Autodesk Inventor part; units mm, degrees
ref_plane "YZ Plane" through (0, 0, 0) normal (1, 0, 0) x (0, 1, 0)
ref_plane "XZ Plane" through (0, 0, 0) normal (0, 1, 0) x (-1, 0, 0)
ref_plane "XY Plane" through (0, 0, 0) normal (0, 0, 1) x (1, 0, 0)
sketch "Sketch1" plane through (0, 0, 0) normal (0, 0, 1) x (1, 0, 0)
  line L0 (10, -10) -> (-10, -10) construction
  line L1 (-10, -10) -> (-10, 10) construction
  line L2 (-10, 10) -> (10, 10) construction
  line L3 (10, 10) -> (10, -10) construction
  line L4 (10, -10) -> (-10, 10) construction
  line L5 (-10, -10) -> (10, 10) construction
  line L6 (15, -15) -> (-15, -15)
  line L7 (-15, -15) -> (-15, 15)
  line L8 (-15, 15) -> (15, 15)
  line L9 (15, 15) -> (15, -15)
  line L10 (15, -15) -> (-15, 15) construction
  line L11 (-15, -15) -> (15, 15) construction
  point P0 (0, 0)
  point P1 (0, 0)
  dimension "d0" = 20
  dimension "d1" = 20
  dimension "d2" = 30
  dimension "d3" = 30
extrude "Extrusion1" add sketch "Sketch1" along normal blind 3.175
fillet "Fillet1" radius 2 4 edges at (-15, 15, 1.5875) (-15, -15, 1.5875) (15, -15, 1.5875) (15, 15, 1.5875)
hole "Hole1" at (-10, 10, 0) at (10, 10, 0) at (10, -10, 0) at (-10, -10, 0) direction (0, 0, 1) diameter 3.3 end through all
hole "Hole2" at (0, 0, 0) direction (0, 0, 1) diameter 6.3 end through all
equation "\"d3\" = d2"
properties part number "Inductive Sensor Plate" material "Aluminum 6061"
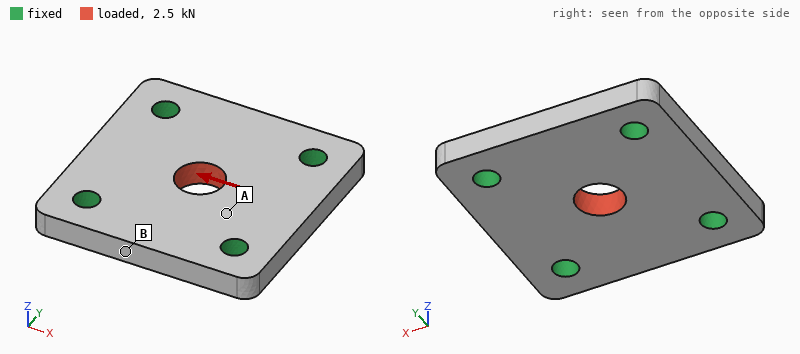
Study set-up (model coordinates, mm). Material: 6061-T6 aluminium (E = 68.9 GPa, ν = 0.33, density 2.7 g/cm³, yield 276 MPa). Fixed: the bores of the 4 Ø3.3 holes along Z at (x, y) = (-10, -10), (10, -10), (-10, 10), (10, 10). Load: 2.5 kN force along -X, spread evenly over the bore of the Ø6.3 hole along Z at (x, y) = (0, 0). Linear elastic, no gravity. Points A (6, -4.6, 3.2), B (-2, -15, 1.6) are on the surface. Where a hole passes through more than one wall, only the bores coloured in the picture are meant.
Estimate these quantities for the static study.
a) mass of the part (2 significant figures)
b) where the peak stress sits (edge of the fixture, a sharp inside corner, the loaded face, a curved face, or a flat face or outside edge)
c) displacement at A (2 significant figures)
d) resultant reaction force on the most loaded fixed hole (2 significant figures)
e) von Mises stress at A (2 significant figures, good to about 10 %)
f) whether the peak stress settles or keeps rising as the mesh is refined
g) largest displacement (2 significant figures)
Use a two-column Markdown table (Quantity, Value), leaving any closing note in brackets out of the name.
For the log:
| Quantity | Value |
|---|---|
| mass of the part | 7.1 g |
| where the peak stress sits | edge of the fixture |
| displacement at A | 3.3 µm |
| resultant reaction force on the most loaded fixed hole | 680 N |
| von Mises stress at A | 30 MPa |
| whether the peak stress settles or keeps rising as the mesh is refined | keeps rising |
| largest displacement | 6.4 µm |
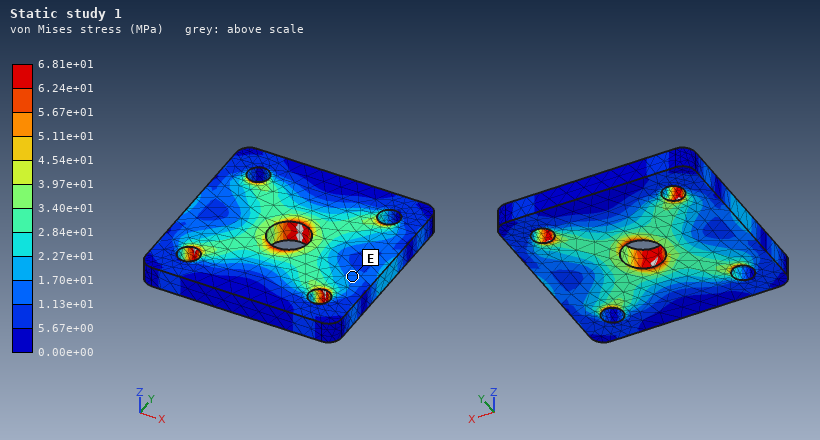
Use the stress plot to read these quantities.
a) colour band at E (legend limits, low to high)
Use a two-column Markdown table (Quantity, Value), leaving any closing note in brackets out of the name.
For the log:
| Quantity | Value |
|---|---|
| colour band at E | 1.13e+01 to 1.70e+01 MPa |
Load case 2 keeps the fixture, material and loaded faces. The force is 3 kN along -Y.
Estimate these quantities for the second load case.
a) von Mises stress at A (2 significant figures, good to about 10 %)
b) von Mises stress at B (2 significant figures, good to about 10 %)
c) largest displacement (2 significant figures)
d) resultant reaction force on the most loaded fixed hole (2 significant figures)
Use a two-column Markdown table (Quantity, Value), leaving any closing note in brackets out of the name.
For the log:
| Quantity | Value |
|---|---|
| von Mises stress at A | 35 MPa |
| von Mises stress at B | 23 MPa |
| largest displacement | 7.7 µm |
| resultant reaction force on the most loaded fixed hole | 820 N |
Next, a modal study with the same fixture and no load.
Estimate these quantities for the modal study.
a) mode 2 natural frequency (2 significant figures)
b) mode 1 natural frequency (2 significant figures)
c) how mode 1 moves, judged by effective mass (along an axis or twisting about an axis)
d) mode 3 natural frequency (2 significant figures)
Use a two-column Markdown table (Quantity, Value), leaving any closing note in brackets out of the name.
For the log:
| Quantity | Value |
|---|---|
| mode 2 natural frequency | 41 kHz |
| mode 1 natural frequency | 31 kHz |
| how mode 1 moves, judged by effective mass | along Z |
| mode 3 natural frequency | 41 kHz |
